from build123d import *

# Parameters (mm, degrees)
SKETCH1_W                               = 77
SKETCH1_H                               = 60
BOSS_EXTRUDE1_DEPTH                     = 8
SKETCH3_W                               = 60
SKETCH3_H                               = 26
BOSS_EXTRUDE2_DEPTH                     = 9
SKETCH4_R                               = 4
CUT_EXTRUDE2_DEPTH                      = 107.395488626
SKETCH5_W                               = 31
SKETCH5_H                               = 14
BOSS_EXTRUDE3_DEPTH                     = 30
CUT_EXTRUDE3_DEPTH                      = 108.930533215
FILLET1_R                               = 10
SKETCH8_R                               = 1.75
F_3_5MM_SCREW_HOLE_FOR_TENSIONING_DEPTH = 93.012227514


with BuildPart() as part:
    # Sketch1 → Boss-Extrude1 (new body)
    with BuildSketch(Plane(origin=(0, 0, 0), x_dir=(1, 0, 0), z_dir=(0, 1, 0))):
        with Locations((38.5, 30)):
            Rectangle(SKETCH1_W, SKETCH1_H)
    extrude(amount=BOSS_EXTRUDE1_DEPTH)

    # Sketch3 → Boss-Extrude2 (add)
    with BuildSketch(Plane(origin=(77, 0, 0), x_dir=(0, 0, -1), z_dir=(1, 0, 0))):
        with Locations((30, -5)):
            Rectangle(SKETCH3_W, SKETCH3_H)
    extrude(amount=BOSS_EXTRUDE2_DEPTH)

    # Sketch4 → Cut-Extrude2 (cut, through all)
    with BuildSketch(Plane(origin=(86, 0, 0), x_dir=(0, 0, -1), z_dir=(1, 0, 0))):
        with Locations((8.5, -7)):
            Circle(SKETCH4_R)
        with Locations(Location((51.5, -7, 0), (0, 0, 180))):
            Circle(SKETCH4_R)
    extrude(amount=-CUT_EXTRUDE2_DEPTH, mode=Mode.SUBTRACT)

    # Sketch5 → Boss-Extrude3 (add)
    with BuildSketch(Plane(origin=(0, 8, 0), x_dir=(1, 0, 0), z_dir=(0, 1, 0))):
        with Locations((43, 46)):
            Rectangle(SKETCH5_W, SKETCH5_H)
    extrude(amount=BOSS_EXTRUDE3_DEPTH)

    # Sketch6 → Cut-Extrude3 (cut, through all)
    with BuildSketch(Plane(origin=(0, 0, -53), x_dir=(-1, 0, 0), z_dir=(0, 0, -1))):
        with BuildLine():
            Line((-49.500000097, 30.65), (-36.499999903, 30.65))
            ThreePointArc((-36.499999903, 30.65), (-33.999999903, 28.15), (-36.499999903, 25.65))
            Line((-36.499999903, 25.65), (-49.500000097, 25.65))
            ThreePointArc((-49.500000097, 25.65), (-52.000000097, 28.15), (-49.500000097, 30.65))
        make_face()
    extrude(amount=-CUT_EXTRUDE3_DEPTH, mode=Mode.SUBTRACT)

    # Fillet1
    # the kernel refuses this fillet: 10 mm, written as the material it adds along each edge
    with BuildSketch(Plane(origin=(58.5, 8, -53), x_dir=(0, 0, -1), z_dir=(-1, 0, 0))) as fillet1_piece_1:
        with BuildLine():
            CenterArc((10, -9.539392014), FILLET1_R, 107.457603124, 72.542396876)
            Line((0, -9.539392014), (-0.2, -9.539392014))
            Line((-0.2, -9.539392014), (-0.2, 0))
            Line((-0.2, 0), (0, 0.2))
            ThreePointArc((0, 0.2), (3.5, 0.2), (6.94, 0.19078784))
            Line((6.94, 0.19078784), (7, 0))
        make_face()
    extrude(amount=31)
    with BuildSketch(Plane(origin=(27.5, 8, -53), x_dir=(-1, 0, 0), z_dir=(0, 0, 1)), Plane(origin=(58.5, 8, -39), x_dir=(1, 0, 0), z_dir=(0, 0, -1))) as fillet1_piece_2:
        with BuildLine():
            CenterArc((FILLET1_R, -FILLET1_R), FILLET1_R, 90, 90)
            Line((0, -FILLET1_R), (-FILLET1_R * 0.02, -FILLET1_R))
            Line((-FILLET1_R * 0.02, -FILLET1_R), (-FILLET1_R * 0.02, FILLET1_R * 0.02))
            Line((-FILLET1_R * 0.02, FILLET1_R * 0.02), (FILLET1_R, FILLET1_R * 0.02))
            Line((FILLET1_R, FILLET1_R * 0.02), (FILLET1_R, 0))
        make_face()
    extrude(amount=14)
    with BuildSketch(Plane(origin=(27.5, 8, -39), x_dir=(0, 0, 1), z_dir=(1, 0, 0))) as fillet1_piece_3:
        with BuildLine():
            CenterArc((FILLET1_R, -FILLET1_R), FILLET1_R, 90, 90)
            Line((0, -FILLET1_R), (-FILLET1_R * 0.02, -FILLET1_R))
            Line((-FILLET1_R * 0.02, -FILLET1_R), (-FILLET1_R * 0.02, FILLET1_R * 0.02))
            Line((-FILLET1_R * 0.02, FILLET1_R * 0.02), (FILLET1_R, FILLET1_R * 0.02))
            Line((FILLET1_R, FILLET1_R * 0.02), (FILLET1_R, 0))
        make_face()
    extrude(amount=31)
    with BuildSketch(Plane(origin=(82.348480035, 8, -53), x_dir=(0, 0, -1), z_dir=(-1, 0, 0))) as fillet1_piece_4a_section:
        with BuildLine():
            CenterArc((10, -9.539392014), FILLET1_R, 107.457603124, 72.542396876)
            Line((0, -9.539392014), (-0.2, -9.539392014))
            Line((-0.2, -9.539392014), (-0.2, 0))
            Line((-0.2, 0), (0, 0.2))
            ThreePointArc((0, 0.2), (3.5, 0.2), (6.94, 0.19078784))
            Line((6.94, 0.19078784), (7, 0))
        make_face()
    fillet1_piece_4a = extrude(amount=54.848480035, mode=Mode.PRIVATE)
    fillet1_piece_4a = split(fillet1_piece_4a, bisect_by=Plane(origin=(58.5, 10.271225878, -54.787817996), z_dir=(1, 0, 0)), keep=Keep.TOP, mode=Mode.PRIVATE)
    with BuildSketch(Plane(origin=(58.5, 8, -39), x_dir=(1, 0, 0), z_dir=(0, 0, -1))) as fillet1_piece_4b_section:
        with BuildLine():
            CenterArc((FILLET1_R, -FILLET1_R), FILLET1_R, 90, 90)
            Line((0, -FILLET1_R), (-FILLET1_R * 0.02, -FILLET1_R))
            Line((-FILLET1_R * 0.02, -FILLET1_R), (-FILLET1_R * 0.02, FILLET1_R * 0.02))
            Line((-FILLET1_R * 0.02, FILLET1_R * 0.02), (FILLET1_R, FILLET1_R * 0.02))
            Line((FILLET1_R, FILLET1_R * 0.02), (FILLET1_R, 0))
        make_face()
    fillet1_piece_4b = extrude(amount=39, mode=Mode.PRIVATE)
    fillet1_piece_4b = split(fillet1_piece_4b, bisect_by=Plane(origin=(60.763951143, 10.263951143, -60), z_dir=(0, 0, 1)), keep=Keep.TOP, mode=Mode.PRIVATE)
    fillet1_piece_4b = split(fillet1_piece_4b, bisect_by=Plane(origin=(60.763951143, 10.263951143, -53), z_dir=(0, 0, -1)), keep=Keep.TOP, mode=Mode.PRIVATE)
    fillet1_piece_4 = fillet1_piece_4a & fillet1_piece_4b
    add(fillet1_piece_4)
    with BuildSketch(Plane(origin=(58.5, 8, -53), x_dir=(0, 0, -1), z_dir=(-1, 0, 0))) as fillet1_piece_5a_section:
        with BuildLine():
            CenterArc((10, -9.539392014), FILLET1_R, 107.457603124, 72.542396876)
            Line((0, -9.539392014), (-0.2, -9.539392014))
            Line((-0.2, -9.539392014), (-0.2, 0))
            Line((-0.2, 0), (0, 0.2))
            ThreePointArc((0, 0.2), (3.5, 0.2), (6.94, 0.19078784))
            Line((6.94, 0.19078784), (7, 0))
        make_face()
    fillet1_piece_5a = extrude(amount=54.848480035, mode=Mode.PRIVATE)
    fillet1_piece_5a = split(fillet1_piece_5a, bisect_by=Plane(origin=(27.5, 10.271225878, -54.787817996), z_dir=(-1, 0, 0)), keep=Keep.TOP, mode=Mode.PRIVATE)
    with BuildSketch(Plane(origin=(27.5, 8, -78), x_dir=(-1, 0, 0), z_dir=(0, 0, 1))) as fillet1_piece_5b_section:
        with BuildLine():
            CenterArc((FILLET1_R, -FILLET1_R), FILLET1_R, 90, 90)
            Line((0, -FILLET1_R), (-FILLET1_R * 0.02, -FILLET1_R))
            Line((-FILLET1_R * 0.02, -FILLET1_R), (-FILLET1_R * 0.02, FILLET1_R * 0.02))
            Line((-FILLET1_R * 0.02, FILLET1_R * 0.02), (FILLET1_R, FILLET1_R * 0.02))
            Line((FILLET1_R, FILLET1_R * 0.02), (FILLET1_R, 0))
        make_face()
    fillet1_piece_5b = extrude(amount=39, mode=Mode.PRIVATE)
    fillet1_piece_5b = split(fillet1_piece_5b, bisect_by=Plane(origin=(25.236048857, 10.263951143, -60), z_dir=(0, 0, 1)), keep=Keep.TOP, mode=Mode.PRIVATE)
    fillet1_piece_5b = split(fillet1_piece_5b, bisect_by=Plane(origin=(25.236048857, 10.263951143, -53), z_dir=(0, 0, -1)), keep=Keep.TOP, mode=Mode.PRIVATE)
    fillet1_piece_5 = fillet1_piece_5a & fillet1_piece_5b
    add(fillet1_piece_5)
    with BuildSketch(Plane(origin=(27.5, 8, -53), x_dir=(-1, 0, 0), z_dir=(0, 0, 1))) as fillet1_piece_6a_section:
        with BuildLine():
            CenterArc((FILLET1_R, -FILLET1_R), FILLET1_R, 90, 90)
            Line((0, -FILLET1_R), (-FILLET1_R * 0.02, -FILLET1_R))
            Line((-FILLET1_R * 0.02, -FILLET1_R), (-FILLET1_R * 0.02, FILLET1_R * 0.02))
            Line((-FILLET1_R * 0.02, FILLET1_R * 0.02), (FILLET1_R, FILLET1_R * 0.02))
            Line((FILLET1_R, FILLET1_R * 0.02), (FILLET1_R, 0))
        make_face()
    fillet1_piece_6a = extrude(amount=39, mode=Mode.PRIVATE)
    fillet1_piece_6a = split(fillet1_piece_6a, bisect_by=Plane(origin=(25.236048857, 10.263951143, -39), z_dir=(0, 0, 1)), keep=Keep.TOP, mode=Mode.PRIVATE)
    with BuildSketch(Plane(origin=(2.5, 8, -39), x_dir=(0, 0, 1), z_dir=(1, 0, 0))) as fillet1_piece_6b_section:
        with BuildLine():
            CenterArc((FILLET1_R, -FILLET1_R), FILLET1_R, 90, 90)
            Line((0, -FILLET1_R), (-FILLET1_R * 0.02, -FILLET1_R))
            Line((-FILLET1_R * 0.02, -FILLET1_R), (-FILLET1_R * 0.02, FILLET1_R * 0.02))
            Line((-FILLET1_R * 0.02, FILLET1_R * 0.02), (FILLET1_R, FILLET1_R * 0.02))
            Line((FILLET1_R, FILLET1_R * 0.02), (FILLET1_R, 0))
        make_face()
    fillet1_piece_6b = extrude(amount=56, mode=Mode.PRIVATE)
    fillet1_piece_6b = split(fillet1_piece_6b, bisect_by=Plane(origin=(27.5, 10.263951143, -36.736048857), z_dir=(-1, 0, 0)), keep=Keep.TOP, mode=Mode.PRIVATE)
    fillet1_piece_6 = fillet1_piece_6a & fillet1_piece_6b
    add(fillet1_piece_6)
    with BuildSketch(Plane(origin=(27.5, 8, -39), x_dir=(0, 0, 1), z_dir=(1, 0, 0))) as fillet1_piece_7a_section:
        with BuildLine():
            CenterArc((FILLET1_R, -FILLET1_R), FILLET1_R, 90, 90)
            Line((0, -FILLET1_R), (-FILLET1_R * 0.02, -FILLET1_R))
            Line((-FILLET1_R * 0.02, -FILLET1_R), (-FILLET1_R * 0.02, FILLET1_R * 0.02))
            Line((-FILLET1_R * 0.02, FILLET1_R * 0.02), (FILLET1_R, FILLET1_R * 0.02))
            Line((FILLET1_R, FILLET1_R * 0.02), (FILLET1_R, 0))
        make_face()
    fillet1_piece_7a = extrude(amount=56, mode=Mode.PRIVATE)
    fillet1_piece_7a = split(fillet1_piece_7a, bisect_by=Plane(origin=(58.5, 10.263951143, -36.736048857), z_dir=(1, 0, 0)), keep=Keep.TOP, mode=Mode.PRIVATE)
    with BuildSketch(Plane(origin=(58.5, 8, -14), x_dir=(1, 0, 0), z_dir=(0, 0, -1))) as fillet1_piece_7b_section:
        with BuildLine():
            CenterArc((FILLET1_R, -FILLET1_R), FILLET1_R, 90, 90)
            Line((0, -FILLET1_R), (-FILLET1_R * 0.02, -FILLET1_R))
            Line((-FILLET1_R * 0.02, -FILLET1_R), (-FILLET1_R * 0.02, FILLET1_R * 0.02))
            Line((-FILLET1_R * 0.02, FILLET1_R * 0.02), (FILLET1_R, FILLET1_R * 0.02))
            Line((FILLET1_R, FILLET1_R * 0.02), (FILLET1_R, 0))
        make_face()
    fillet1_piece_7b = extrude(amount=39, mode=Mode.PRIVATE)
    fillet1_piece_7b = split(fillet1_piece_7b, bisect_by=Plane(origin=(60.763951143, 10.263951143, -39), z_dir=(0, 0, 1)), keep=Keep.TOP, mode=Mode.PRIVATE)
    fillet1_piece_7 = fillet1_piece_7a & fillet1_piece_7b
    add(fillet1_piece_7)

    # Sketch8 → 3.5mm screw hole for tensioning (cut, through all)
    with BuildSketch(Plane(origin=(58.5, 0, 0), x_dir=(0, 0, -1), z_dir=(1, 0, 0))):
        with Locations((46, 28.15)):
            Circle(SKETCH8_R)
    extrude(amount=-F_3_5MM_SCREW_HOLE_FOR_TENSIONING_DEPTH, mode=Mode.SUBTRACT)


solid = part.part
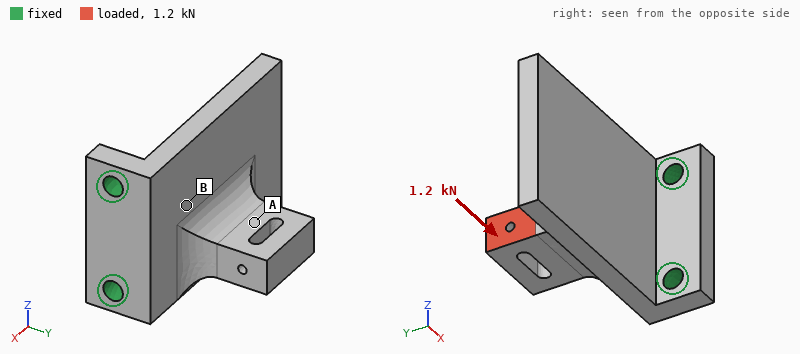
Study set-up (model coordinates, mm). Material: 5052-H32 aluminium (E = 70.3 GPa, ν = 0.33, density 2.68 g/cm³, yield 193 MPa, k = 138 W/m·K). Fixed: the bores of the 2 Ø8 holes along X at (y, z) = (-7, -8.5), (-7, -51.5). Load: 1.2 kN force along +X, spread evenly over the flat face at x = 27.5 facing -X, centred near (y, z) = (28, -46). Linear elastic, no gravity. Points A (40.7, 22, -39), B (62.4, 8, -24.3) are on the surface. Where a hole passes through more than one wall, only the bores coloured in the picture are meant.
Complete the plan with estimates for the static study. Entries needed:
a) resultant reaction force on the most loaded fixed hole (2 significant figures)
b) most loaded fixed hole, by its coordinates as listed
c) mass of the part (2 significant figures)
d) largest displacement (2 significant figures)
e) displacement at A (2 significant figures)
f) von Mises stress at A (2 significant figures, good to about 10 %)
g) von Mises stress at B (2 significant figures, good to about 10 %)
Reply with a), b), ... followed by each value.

a) 1.0 kN
b) (-7, -51.5)
c) 170 g
d) 0.39 mm
e) 0.19 mm
f) 9.4 MPa
g) 30 MPa
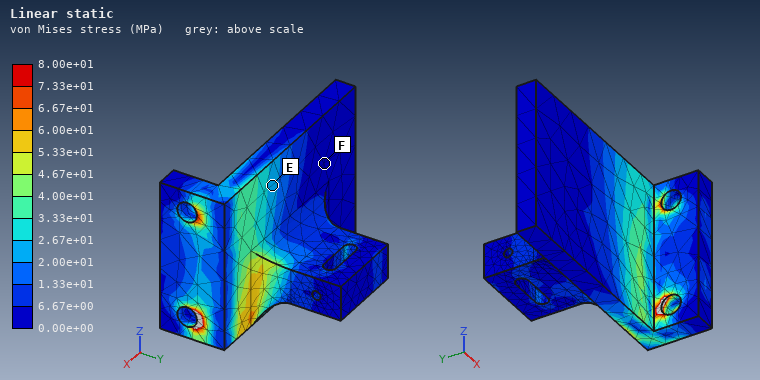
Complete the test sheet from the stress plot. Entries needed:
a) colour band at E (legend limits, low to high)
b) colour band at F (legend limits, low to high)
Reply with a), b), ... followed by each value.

a) 2.00e+01 to 2.67e+01 MPa
b) 0.00e+00 to 6.67e+00 MPa
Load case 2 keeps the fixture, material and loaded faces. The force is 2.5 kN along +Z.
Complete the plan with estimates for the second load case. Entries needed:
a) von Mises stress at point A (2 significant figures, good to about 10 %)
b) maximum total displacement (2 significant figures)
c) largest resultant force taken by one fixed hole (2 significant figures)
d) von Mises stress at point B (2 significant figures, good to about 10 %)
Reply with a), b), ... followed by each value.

a) 42 MPa
b) 0.22 mm
c) 3.8 kN
d) 43 MPa
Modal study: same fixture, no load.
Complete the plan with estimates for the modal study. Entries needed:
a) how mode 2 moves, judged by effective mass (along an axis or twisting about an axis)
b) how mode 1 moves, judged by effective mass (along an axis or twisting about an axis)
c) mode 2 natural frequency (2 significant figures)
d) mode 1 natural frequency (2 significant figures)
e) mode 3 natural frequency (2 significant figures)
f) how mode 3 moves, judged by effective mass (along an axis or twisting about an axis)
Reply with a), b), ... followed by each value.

a) twisting about X
b) along Y
c) 2900 Hz
d) 850 Hz
e) 3600 Hz
f) along Z
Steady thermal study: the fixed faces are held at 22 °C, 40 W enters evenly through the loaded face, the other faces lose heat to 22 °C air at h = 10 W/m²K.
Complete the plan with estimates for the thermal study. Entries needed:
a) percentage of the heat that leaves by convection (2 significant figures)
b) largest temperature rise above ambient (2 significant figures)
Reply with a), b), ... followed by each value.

a) 8.2 %
b) 52 K
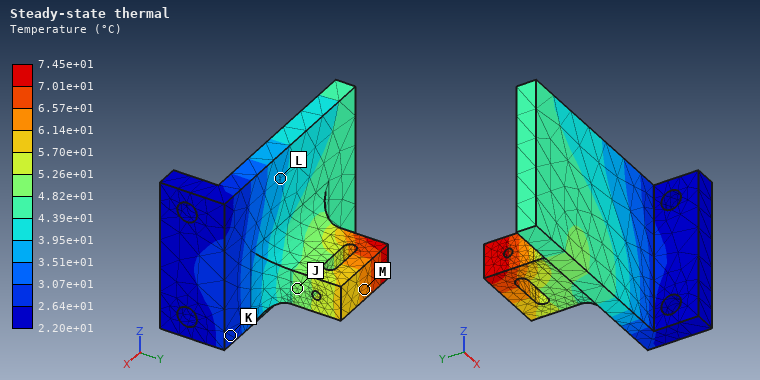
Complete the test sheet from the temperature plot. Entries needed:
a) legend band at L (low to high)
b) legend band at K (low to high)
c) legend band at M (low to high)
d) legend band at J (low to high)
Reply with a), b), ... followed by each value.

a) 3.51e+01 to 3.95e+01 °C
b) 2.64e+01 to 3.07e+01 °C
c) 6.14e+01 to 6.57e+01 °C
d) 4.82e+01 to 5.26e+01 °C
